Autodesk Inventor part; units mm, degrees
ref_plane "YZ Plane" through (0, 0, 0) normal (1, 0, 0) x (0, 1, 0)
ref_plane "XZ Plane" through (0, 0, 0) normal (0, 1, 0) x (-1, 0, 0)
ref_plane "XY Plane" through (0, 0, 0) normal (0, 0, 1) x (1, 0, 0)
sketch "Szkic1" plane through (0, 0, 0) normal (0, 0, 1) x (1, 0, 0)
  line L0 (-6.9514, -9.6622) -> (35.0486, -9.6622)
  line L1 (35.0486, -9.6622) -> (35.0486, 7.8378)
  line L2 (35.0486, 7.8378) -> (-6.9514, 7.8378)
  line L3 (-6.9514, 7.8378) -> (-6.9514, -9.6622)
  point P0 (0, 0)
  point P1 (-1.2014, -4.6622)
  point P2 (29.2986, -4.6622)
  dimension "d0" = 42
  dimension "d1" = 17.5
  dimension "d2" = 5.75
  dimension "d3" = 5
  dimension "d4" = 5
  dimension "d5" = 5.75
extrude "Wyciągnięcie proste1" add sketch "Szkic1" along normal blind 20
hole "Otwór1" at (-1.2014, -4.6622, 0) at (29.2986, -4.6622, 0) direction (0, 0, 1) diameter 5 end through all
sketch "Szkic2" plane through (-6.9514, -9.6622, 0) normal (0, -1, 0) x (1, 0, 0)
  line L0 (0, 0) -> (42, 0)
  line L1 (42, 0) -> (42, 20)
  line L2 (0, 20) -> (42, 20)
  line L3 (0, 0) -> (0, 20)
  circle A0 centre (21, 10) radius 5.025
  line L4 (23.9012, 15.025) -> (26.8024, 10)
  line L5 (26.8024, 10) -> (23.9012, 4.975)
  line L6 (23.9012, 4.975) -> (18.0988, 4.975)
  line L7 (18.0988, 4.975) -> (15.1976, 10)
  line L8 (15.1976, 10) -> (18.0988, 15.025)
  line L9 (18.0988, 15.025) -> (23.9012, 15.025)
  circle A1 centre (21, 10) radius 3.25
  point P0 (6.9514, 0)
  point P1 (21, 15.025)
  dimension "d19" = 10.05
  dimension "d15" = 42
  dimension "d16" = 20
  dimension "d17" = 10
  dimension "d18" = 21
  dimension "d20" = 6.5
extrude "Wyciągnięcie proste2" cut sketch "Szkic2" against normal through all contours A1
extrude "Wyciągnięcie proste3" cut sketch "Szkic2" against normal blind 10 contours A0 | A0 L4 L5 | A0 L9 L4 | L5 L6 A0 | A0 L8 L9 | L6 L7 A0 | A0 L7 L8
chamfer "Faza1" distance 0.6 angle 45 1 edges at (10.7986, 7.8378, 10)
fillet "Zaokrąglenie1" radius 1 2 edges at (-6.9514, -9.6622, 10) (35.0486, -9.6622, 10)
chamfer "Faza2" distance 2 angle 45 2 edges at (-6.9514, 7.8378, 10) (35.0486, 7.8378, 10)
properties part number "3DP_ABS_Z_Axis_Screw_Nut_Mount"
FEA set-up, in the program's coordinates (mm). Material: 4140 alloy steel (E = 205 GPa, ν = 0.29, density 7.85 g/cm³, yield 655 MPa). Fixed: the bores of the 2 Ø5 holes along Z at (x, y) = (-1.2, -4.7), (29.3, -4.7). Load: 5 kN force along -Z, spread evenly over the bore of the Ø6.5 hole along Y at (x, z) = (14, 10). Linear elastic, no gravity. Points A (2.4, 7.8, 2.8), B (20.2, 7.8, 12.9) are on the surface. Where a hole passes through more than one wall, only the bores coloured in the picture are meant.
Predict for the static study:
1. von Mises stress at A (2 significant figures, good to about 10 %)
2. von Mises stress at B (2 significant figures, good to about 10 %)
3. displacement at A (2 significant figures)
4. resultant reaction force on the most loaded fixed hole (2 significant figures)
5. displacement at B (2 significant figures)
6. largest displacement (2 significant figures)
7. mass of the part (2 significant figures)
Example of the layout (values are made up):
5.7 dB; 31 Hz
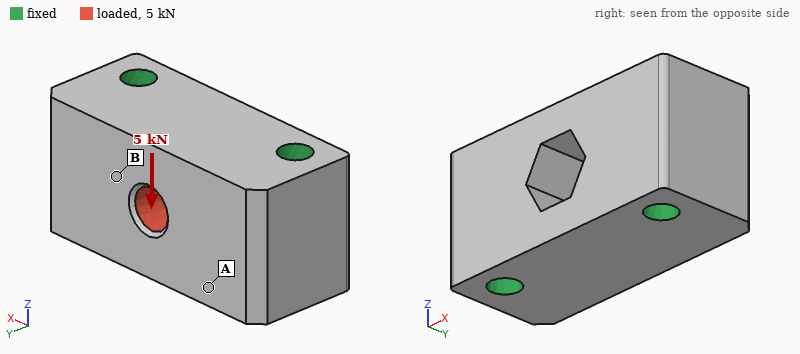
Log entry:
12 MPa; 26 MPa; 1.7 µm; 2.5 kN; 2.7 µm; 3.9 µm; 100 g
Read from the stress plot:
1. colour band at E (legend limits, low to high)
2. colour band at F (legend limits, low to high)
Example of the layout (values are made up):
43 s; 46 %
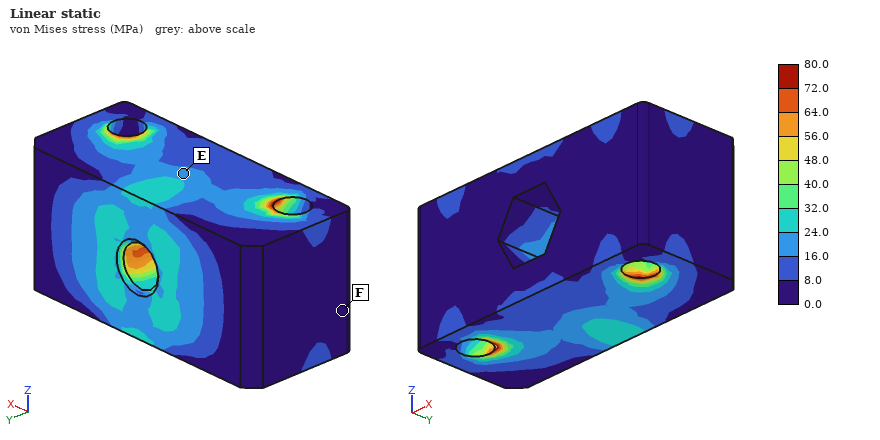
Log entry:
16.0 to 24.0 MPa; 0.0 to 8.0 MPa
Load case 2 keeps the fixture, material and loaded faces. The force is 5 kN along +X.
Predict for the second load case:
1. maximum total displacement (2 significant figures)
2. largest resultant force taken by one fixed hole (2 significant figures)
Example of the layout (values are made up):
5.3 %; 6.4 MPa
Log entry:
1.8 µm; 2.7 kN
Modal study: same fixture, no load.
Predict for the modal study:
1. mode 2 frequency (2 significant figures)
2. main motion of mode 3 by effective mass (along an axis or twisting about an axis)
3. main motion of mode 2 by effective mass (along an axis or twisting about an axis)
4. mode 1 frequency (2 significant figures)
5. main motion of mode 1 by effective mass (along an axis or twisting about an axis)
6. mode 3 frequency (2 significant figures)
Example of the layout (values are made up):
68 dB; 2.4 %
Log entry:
41 kHz; along X; along Y; 39 kHz; along Z; 51 kHz
